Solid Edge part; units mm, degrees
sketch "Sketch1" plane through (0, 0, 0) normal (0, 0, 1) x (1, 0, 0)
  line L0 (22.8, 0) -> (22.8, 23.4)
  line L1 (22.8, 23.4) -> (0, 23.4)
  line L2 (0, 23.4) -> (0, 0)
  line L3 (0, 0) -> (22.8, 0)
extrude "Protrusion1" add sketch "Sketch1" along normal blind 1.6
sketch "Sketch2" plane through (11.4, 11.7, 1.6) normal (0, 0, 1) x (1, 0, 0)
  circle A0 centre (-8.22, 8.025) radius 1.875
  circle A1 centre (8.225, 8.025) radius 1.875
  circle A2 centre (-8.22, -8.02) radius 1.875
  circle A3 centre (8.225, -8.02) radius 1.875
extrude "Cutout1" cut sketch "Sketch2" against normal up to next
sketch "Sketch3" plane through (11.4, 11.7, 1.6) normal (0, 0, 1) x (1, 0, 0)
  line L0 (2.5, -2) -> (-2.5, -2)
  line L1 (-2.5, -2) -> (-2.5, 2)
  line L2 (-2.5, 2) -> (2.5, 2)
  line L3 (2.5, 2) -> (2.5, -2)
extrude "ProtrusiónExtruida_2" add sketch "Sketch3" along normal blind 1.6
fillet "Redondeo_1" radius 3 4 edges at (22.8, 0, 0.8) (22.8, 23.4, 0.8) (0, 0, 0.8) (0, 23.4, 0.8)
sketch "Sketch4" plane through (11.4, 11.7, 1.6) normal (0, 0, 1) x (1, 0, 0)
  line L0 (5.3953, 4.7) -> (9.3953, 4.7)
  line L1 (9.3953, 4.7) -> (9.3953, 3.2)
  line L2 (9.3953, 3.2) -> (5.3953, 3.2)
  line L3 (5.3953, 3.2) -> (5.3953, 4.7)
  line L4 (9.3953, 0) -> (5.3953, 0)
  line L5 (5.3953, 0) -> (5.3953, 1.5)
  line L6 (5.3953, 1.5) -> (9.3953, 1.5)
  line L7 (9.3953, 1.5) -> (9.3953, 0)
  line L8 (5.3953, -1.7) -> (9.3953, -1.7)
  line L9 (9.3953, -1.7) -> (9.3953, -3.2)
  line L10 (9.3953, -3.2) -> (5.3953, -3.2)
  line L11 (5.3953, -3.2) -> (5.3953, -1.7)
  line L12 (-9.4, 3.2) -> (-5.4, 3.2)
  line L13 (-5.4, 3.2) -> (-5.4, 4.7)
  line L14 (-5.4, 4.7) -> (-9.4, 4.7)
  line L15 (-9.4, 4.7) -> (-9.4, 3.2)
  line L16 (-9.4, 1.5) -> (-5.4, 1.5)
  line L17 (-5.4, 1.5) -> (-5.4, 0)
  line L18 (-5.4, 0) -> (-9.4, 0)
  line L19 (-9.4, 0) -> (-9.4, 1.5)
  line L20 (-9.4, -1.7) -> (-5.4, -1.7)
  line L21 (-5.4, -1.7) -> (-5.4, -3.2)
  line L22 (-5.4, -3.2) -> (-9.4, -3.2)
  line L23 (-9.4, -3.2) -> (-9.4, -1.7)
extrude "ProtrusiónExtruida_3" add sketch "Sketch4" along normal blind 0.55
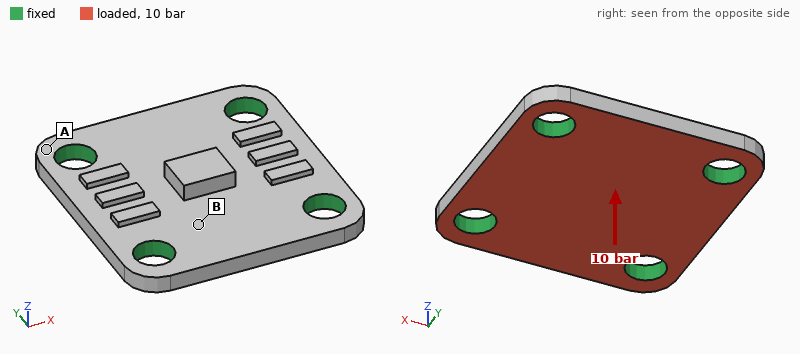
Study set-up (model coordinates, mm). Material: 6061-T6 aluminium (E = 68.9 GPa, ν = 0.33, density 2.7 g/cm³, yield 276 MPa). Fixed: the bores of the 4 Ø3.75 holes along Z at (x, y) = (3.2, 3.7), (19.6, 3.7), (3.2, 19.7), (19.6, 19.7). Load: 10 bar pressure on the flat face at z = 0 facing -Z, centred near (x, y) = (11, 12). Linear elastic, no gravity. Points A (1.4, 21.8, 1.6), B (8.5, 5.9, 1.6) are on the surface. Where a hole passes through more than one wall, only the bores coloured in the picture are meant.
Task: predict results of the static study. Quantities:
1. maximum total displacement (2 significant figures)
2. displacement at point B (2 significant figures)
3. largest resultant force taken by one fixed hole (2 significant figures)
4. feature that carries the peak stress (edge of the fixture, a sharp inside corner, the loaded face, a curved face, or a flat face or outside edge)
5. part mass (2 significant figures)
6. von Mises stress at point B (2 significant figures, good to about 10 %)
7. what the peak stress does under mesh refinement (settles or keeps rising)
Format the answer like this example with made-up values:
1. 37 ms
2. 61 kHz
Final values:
1. 8.4 µm
2. 5.0 µm
3. 120 N
4. edge of the fixture
5. 2.2 g
6. 13 MPa
7. keeps rising
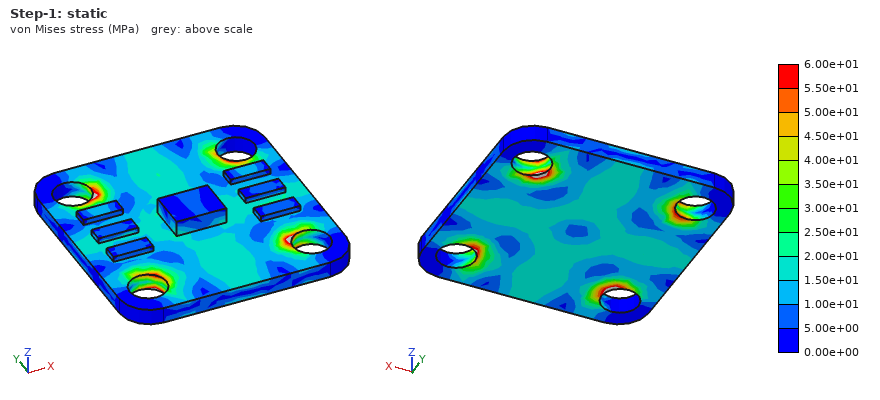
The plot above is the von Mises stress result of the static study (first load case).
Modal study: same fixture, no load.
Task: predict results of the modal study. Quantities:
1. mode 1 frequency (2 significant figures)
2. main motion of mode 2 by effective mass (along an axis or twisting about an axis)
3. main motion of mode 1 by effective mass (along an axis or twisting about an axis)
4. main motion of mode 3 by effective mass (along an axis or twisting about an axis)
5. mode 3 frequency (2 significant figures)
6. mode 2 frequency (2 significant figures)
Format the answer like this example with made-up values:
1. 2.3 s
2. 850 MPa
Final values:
1. 29 kHz
2. twisting about X
3. along Z
4. twisting about Y
5. 45 kHz
6. 43 kHz
